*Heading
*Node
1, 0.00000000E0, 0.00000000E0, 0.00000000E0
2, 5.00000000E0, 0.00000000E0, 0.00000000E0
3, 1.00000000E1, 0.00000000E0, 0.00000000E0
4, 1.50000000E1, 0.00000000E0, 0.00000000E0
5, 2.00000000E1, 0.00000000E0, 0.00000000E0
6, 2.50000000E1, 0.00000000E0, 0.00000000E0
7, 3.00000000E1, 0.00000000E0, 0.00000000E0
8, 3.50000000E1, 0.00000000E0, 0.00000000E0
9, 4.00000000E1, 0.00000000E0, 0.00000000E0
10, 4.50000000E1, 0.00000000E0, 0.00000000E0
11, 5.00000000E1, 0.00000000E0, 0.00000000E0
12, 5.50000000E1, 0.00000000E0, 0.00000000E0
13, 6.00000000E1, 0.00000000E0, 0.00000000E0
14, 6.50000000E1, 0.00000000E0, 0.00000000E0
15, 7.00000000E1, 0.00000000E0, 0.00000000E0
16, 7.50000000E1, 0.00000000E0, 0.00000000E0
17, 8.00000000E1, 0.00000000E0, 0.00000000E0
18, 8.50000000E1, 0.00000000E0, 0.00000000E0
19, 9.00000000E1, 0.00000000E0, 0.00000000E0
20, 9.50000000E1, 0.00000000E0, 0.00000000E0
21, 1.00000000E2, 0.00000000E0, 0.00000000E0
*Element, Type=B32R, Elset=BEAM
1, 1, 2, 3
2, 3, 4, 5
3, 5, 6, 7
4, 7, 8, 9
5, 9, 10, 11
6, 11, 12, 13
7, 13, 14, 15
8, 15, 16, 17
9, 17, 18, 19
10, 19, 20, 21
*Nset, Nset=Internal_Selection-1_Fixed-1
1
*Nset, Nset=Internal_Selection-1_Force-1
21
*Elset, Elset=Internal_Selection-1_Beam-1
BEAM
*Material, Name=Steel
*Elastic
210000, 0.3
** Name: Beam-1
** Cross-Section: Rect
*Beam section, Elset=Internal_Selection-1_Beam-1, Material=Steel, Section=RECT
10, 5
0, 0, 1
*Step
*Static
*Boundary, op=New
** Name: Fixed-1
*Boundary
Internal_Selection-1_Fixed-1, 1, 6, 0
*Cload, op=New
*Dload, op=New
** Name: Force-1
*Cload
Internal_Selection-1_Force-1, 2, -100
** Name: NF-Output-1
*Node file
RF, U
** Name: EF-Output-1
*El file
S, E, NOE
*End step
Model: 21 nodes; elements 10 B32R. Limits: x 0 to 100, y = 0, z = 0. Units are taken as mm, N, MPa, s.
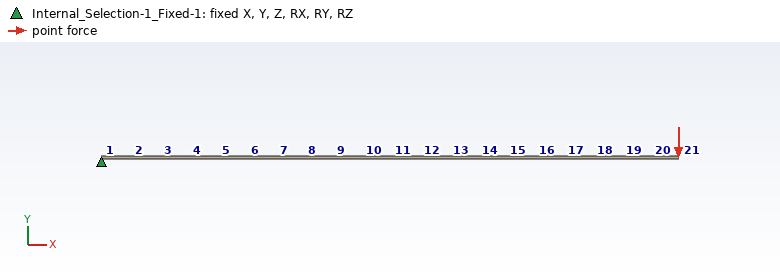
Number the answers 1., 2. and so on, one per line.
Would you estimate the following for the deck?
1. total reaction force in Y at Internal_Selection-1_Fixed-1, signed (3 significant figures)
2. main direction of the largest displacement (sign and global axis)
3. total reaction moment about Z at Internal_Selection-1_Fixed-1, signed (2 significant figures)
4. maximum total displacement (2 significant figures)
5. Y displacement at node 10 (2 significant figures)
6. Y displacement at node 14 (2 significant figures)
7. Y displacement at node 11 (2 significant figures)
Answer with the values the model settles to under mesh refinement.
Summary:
1. 100 N
2. -Y
3. 10000 N·mm
4. 1.5 mm
5. -0.39 mm
6. -0.76 mm
7. -0.48 mm
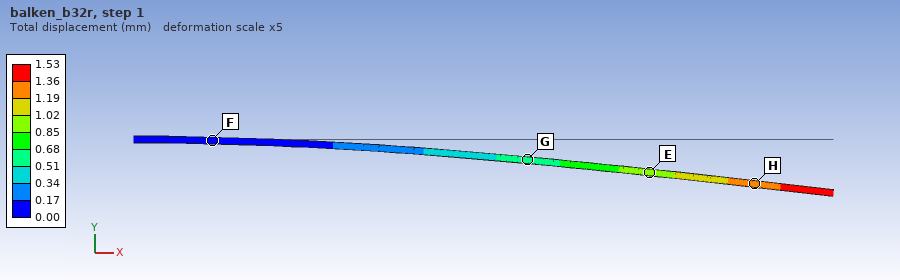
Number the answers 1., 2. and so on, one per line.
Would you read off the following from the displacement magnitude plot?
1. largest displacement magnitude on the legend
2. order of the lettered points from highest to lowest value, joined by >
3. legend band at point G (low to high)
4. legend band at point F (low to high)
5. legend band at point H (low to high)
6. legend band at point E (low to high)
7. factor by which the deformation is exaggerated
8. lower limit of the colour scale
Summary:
1. 1.53 mm
2. H > E > G > F
3. 0.51 to 0.68 mm
4. 0.00 to 0.17 mm
5. 1.19 to 1.36 mm
6. 0.85 to 1.02 mm
7. 5
8. 0.00 mm
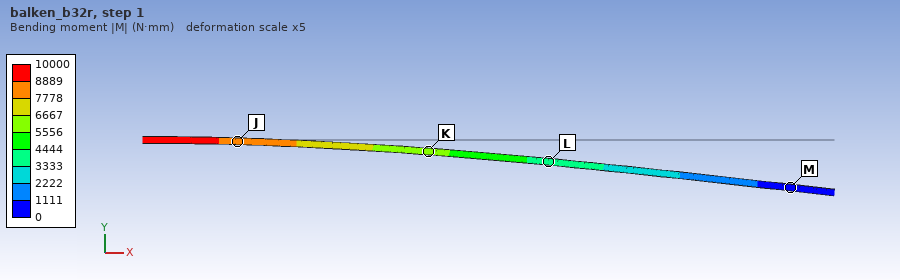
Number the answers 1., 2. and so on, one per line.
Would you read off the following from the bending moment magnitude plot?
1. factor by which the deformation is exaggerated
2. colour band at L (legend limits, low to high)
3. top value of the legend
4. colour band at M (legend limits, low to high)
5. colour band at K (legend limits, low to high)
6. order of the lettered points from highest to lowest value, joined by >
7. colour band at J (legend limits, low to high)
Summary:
1. 5
2. 3333 to 4444 N·mm
3. 10000 N·mm
4. 0 to 1111 N·mm
5. 5556 to 6667 N·mm
6. J > K > L > M
7. 7778 to 8889 N·mm
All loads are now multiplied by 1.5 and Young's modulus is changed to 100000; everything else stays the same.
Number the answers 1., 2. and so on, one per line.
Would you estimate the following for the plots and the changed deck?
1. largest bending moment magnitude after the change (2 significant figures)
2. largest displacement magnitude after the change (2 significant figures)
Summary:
1. 15000 N·mm
2. 4.8 mm
